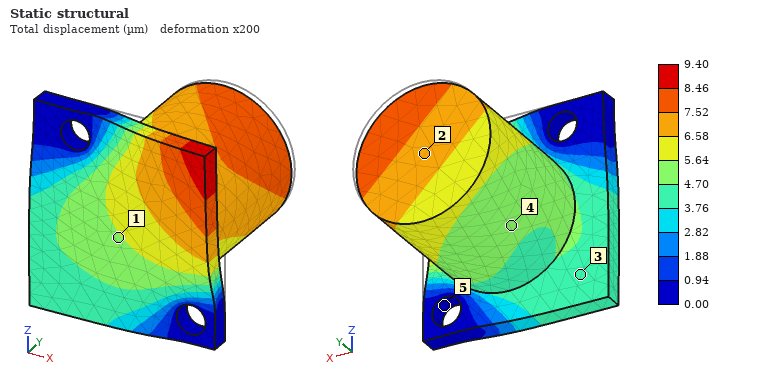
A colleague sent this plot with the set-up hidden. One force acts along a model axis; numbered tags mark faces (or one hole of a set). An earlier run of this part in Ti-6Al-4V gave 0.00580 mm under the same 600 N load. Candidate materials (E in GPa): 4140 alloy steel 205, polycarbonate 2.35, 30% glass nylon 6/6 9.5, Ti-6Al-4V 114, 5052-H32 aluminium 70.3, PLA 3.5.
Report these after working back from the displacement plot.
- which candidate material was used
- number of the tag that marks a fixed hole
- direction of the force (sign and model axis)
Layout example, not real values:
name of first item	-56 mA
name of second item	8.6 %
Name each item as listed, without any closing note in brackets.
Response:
which candidate material was used	5052-H32 aluminium
number of the tag that marks a fixed hole	5
direction of the force	-Y
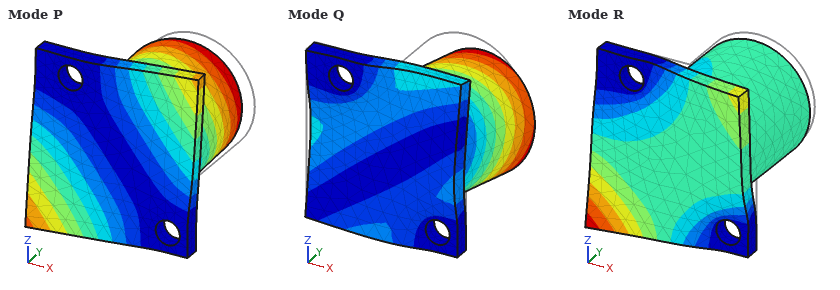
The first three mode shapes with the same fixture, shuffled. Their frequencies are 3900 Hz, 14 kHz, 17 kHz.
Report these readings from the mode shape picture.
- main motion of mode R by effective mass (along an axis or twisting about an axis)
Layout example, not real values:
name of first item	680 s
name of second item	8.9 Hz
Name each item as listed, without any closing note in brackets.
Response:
main motion of mode R by effective mass	along Y
